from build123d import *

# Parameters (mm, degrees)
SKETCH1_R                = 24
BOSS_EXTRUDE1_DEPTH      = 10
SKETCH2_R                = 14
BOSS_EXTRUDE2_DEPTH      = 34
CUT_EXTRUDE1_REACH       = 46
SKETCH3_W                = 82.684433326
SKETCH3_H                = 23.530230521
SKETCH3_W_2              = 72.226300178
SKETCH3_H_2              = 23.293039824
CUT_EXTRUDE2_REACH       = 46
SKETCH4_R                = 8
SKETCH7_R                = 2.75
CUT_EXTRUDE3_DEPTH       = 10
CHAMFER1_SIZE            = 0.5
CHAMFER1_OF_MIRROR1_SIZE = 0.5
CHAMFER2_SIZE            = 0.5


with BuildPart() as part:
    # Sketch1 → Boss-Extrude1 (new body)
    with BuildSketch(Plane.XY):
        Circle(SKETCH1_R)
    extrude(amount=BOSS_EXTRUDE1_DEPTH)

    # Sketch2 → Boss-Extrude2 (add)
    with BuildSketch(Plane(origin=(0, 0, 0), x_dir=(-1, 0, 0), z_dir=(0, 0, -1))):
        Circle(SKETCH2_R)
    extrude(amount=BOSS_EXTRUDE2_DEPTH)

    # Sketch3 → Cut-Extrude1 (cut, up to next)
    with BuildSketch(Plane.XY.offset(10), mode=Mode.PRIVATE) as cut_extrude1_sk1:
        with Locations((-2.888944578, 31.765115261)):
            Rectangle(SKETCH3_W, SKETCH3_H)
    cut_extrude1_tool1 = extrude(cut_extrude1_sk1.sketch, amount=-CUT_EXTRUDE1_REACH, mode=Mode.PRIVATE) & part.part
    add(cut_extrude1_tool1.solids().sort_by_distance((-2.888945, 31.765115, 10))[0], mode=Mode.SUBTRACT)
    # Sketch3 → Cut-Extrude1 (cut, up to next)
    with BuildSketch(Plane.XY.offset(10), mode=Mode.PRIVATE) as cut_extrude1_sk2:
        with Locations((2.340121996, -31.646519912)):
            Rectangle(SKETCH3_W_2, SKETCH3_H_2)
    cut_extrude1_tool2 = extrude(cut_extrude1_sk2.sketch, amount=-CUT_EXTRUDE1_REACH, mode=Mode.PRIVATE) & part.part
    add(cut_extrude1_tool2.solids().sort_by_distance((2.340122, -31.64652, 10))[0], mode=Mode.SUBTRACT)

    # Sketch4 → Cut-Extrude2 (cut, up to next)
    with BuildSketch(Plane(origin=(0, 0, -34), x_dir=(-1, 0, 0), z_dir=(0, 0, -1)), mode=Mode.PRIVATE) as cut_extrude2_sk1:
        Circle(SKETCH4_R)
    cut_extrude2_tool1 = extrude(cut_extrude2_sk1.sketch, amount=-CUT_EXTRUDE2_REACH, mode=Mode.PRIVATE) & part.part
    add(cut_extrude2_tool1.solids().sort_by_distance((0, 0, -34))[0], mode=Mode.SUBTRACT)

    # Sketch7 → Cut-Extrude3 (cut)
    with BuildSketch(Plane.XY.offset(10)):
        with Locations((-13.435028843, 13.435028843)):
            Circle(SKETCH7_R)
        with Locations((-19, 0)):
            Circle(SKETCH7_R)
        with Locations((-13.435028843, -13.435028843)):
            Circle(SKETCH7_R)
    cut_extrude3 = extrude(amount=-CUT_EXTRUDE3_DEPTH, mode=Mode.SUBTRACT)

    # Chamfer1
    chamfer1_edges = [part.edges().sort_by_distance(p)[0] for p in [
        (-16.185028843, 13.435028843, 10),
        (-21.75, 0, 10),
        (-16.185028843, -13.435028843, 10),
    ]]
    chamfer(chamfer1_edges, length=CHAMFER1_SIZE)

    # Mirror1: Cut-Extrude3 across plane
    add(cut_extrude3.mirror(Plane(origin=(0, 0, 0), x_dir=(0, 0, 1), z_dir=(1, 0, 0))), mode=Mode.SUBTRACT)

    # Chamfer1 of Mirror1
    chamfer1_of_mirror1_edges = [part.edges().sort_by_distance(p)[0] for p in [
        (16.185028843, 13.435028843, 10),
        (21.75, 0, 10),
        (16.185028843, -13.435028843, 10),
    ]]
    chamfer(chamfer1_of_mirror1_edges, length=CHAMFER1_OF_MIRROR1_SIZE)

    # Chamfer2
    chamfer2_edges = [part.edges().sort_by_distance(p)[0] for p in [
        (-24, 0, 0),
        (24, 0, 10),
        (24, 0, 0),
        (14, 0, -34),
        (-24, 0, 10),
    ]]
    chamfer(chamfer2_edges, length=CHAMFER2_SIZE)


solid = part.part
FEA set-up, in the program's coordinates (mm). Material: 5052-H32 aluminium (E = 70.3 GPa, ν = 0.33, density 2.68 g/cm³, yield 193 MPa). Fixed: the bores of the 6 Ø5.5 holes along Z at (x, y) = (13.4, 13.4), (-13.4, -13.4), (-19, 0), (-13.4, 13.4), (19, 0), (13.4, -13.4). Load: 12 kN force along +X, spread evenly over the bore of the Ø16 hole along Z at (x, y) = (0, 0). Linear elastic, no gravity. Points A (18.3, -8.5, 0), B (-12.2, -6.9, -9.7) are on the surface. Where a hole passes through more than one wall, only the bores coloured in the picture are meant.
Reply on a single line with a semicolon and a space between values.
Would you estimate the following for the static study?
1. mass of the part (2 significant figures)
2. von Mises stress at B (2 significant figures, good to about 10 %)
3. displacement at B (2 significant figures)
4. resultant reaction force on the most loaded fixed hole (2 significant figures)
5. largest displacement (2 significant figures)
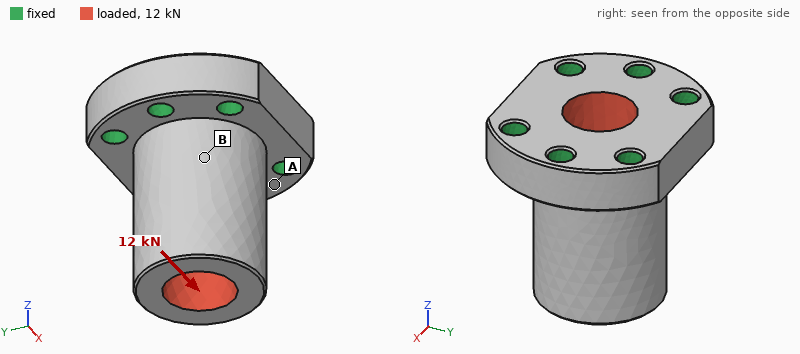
73 g; 36 MPa; 27 µm; 3.9 kN; 71 µm
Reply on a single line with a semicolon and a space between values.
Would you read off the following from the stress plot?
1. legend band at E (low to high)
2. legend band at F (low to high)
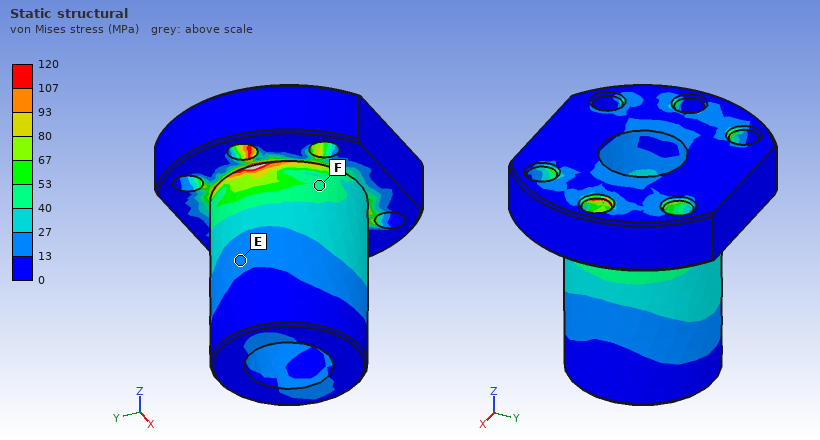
13 to 27 MPa; 40 to 53 MPa
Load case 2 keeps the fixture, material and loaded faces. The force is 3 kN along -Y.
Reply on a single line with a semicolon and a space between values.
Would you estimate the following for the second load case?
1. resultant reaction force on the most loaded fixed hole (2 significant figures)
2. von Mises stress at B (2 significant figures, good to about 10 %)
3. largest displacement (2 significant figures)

1.2 kN; 9.2 MPa; 21 µm
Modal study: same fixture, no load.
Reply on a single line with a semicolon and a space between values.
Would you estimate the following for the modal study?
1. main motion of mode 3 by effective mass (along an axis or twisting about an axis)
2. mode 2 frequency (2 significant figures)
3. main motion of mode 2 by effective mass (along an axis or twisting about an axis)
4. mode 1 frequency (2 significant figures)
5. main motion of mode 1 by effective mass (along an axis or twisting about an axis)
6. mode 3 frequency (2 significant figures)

twisting about Z; 11 kHz; along X; 10 kHz; along Y; 21 kHz
